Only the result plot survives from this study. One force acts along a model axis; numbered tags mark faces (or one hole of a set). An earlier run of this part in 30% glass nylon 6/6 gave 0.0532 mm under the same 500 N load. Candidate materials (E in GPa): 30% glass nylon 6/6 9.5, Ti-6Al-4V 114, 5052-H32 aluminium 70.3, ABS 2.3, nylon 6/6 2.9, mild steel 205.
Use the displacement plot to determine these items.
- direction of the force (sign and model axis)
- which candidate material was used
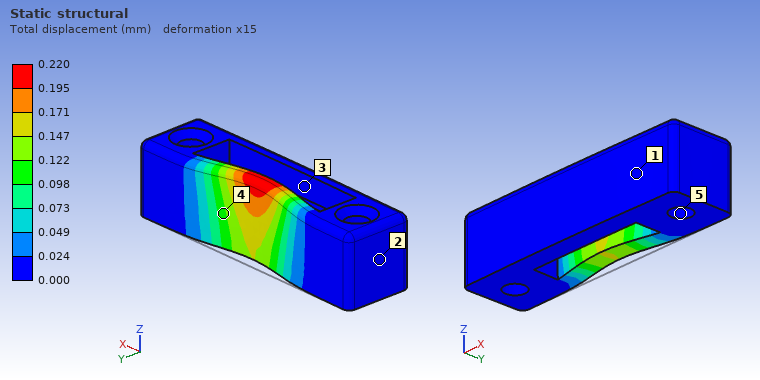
-Y
ABS
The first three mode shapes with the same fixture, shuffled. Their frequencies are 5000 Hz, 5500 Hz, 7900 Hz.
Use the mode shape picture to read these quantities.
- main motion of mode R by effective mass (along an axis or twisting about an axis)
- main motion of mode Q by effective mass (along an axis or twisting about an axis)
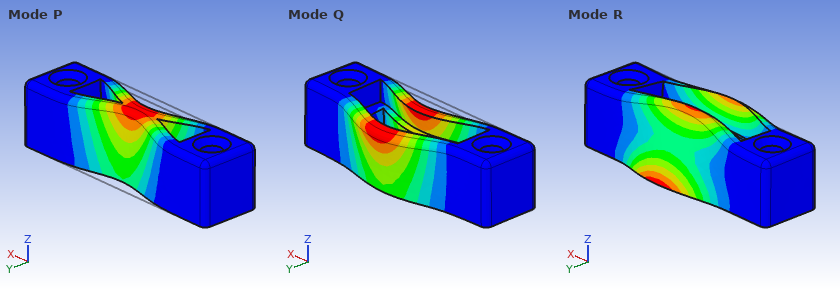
twisting about X
along Y
